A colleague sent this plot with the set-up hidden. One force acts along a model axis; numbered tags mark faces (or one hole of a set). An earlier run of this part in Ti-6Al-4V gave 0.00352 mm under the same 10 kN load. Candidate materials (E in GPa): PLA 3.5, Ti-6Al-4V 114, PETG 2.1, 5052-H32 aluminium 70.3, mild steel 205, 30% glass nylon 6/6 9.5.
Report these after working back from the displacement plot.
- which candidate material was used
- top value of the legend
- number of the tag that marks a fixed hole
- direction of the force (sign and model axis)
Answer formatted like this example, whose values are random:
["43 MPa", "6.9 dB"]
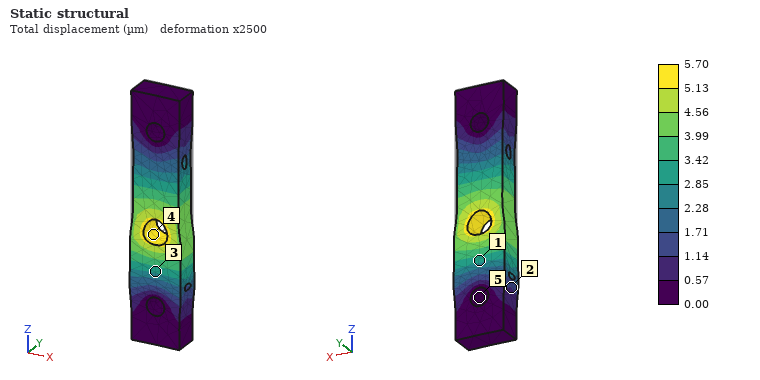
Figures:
["5052-H32 aluminium", "5.70 µm", "5", "-Z"]
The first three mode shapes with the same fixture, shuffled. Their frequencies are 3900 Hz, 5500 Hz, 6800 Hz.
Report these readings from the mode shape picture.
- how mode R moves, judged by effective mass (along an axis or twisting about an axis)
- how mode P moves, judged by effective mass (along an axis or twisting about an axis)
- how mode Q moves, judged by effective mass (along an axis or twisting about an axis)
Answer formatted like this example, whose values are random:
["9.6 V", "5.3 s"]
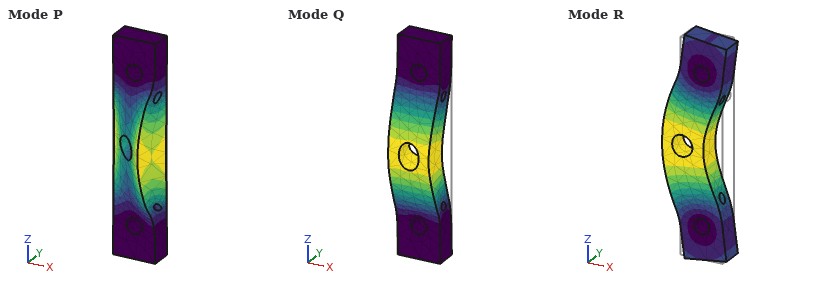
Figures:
["along X", "twisting about Z", "along Y"]
